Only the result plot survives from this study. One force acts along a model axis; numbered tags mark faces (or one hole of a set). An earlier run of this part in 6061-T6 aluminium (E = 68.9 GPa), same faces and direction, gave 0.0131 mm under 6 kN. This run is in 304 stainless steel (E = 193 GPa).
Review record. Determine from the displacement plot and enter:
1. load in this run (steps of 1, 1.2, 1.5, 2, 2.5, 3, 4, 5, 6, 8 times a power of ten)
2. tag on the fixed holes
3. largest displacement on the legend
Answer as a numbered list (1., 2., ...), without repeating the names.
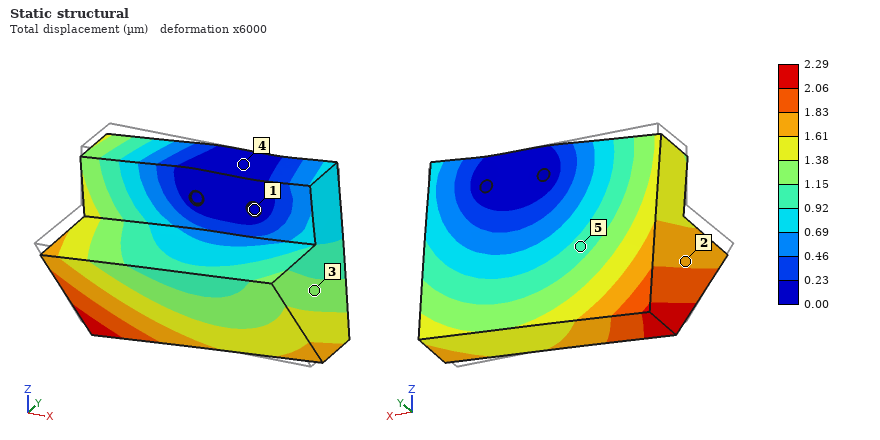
1. 3 kN
2. 1
3. 2.29 µm
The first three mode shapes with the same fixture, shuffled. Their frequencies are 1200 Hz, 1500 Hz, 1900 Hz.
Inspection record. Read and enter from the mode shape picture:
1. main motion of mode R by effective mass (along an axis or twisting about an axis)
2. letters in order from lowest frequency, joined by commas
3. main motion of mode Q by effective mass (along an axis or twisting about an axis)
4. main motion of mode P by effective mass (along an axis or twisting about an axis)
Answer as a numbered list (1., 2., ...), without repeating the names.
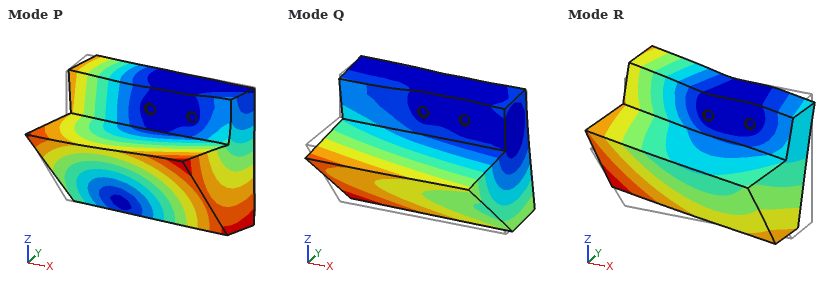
1. along X
2. Q, R, P
3. along Y
4. twisting about Z
